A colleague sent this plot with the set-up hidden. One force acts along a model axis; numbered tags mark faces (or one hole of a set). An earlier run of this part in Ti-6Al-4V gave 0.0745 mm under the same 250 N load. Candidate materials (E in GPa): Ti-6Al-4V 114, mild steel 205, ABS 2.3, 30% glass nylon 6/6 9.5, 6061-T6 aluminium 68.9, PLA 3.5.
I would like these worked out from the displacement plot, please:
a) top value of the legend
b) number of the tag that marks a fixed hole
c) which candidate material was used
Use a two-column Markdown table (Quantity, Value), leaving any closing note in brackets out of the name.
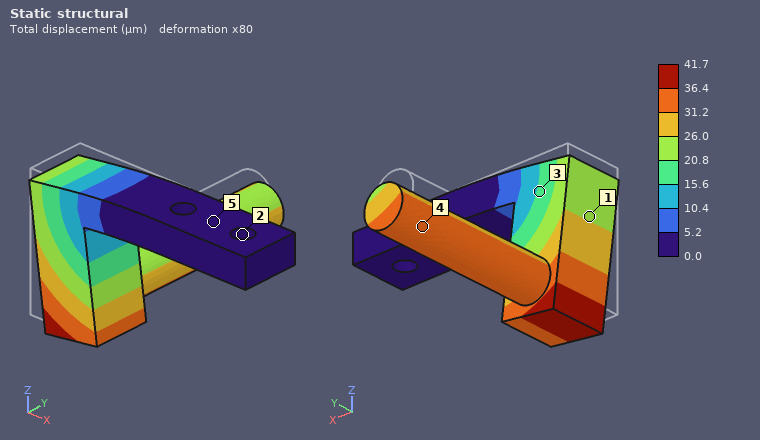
| Quantity | Value |
|---|---|
| top value of the legend | 41.7 µm |
| number of the tag that marks a fixed hole | 2 |
| which candidate material was used | mild steel |
